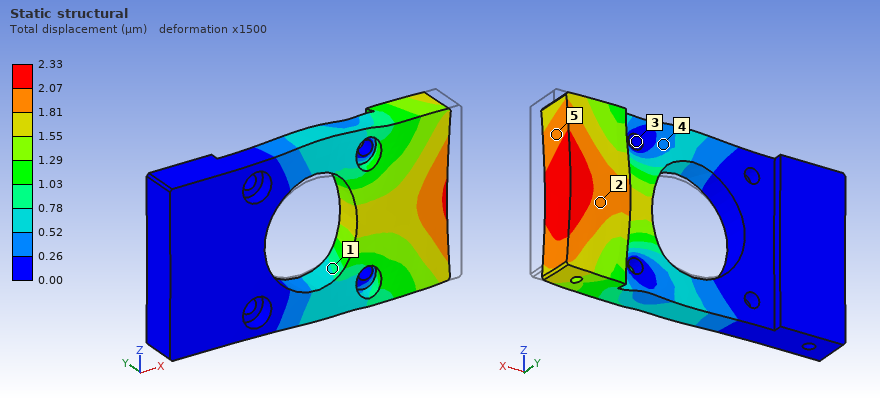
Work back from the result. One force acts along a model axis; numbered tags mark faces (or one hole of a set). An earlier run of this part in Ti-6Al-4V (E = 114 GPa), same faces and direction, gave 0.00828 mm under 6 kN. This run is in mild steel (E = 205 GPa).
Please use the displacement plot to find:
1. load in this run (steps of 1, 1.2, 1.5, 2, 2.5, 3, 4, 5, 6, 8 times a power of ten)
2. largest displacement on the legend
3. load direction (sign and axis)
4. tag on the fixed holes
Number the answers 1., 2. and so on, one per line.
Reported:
1. 3 kN
2. 2.33 µm
3. -X
4. 3
